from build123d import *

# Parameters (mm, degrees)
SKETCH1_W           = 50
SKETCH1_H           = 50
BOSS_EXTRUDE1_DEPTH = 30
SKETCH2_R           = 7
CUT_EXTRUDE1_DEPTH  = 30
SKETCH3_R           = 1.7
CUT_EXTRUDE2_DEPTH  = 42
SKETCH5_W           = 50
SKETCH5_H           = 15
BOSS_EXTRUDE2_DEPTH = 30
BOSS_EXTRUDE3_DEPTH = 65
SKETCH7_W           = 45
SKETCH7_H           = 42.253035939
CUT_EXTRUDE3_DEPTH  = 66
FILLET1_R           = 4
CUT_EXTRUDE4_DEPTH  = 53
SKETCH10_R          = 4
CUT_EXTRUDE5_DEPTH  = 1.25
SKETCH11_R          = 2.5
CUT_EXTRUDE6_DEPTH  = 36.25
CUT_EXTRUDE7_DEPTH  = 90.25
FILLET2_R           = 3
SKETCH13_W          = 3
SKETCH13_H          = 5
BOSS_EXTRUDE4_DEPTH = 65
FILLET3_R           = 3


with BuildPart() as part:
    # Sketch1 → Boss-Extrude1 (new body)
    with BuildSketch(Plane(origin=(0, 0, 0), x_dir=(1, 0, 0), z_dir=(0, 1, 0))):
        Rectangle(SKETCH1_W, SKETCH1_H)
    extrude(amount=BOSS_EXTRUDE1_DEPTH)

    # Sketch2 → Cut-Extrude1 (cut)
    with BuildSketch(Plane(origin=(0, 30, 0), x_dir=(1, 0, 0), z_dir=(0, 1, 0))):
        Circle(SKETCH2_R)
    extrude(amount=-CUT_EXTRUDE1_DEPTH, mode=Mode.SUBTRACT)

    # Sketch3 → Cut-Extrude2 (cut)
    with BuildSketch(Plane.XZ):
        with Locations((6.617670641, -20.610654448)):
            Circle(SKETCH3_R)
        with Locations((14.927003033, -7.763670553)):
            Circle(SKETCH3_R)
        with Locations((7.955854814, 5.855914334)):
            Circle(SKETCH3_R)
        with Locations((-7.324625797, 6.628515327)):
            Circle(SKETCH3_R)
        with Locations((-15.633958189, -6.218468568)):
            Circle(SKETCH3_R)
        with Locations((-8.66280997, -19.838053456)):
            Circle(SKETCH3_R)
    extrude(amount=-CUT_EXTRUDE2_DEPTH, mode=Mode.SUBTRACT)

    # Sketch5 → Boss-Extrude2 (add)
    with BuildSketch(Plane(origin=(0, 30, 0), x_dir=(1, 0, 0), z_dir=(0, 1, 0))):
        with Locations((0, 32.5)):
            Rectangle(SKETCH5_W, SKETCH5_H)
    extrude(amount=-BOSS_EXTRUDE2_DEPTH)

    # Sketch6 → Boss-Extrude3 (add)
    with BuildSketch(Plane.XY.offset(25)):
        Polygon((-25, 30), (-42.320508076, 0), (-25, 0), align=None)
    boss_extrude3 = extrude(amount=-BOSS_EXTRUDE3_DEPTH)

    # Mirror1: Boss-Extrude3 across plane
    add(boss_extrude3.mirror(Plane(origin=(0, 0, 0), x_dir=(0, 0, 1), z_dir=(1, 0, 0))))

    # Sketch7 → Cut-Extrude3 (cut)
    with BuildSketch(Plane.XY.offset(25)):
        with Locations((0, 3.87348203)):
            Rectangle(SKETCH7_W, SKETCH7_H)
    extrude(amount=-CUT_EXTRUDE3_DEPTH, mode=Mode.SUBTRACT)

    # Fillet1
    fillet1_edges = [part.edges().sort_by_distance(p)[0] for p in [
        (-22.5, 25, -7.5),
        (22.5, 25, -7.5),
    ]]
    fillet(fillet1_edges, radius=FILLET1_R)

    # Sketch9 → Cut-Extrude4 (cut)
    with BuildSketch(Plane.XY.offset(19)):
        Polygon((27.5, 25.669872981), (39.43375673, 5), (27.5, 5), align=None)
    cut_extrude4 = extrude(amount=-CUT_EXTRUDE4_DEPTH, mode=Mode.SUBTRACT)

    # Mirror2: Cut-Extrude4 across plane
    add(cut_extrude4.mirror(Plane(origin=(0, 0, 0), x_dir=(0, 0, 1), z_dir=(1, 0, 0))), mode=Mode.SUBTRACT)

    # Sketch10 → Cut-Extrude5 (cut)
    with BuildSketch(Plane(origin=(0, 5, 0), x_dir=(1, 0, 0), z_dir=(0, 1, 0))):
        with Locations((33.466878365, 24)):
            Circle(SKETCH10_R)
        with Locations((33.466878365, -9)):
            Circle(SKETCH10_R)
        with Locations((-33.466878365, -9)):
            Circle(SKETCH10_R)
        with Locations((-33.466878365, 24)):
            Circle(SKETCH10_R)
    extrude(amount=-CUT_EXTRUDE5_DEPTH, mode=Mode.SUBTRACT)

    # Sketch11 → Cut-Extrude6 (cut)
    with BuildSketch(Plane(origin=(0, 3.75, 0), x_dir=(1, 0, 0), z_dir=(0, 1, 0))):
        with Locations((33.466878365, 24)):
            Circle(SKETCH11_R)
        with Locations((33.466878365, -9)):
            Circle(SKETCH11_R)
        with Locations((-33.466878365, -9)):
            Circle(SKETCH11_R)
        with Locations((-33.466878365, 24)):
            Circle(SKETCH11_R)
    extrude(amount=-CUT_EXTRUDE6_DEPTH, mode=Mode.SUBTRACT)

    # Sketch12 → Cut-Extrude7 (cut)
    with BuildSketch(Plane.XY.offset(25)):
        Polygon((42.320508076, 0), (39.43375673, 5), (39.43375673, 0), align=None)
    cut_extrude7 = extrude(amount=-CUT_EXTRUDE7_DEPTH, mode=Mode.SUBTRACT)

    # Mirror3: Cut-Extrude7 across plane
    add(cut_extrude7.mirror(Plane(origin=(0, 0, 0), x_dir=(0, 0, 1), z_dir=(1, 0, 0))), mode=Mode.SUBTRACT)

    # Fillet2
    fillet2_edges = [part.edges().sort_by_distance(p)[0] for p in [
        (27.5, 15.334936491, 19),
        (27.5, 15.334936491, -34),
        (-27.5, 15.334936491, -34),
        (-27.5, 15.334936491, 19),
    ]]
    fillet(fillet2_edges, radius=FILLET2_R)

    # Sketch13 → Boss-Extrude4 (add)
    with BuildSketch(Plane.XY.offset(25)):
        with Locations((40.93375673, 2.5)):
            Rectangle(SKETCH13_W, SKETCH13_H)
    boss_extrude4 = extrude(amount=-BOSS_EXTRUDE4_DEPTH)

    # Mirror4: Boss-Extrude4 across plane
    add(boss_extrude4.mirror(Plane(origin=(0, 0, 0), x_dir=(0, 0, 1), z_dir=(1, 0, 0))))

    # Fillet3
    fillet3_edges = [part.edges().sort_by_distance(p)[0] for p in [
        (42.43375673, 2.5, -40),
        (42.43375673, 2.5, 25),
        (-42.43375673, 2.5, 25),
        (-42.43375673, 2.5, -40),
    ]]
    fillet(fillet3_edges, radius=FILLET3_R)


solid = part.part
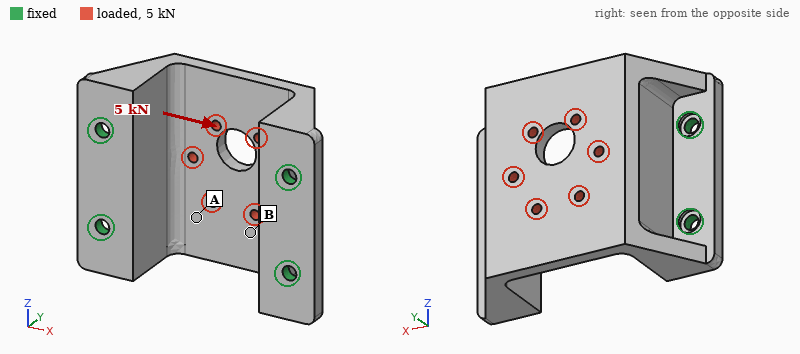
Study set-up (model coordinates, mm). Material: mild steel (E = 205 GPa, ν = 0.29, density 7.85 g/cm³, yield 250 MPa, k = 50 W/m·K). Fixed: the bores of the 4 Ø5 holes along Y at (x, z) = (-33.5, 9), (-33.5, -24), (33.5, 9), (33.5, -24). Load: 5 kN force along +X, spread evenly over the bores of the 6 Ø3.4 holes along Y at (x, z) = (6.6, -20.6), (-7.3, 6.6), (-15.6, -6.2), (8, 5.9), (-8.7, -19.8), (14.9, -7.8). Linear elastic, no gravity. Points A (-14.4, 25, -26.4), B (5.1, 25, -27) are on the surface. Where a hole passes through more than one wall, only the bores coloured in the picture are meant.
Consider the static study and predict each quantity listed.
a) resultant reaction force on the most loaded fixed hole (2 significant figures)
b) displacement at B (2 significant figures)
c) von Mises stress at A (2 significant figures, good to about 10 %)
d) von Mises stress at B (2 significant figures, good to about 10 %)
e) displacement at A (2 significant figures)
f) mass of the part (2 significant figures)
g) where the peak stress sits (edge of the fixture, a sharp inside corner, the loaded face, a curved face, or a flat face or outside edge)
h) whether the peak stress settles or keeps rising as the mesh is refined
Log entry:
1.4 kN
46 µm
70 MPa
29 MPa
45 µm
350 g
edge of the fixture
keeps rising
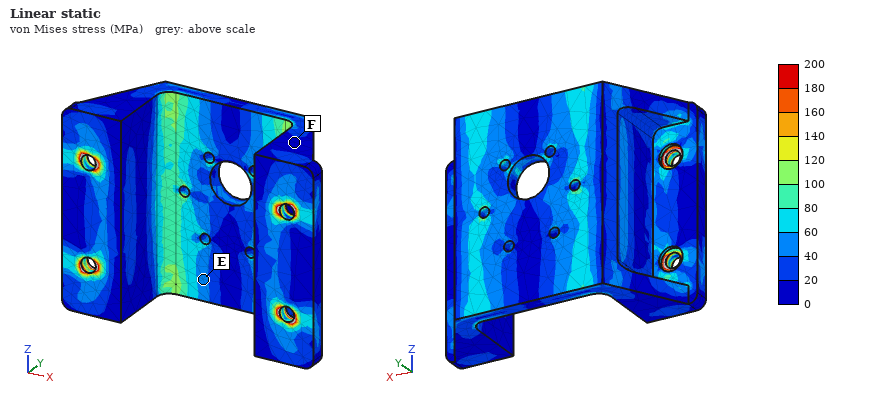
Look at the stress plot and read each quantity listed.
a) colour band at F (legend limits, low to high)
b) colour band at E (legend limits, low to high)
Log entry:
0 to 20 MPa
40 to 60 MPa
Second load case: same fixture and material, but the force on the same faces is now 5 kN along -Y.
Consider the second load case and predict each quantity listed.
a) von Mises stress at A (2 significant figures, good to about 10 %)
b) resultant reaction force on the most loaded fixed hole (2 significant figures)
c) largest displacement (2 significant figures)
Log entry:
32 MPa
1.6 kN
31 µm
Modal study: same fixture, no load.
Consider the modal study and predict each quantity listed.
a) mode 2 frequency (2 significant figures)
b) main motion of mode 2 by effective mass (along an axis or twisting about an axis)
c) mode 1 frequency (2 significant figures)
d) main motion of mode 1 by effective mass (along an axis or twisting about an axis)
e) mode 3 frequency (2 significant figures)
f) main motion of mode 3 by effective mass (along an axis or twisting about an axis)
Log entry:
5900 Hz
twisting about Y
3900 Hz
along X
6200 Hz
along Z
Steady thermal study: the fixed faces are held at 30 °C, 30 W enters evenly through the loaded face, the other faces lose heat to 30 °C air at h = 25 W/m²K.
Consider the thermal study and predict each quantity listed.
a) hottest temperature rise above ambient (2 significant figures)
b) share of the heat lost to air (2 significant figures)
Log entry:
40 K
26 %
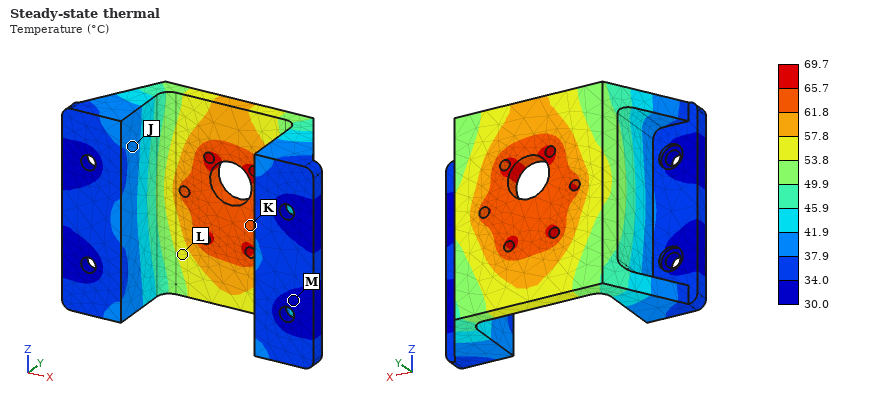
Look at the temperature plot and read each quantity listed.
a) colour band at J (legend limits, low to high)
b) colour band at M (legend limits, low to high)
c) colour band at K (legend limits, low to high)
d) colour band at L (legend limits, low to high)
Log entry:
37.9 to 41.9 °C
30.0 to 34.0 °C
61.8 to 65.7 °C
53.8 to 57.8 °C
